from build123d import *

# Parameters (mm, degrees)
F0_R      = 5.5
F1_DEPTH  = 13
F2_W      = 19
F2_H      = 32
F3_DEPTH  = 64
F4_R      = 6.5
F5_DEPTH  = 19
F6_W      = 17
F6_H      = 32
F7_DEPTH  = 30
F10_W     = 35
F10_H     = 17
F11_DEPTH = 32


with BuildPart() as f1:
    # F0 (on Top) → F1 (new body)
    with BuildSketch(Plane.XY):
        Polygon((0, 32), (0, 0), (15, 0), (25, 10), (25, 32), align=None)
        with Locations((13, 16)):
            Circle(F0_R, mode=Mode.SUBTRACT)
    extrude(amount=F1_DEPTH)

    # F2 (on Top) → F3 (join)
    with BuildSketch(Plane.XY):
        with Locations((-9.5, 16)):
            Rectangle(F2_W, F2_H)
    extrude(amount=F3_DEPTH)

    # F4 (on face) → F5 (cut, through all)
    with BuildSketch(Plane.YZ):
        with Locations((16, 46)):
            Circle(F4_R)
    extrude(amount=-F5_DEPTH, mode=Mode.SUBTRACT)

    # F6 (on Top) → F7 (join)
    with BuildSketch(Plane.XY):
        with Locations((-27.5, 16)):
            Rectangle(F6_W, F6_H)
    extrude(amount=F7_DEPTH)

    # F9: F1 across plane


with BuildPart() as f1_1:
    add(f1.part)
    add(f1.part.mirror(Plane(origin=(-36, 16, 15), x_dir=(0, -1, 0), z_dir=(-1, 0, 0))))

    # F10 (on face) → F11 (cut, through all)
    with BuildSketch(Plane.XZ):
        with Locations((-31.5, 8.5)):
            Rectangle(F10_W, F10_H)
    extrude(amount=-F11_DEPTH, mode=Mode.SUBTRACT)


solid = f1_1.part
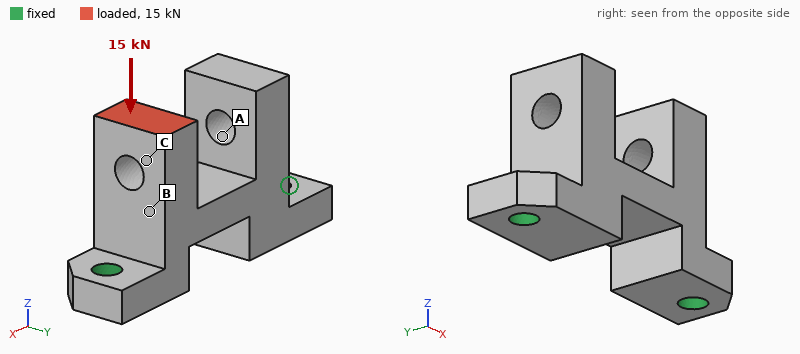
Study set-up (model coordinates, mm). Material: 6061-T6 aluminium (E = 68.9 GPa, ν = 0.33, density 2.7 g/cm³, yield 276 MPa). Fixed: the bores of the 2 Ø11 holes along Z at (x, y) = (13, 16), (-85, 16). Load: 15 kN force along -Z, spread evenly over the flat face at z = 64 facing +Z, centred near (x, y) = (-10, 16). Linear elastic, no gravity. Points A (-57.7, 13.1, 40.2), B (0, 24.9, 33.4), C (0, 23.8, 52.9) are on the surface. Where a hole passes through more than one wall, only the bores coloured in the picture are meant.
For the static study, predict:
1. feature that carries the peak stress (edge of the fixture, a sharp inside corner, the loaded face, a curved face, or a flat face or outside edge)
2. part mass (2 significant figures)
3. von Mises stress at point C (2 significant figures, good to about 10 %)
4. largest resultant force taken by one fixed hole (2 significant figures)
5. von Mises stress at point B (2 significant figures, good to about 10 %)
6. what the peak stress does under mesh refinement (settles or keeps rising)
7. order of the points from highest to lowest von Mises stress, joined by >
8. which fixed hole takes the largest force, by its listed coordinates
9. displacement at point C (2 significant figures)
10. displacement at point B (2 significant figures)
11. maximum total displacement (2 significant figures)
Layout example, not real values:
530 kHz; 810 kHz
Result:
edge of the fixture; 280 g; 49 MPa; 14 kN; 34 MPa; keeps rising; C > B > A; (13, 16); 61 µm; 50 µm; 69 µm
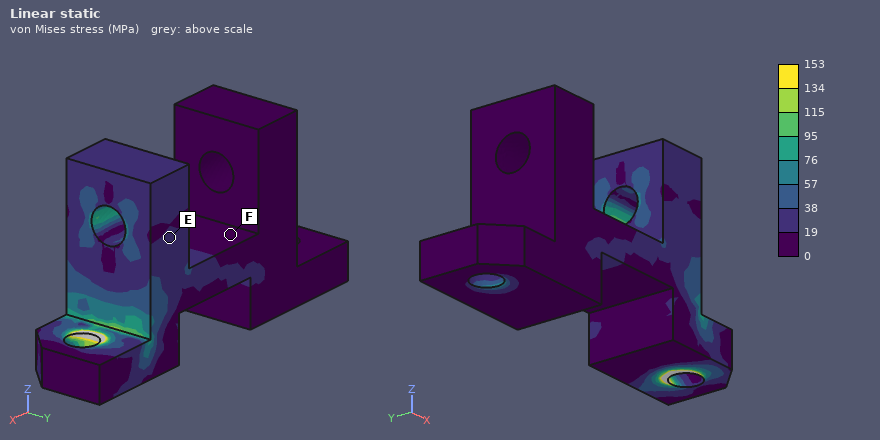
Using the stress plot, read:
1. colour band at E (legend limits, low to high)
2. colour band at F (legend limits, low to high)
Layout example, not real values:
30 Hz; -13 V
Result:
19 to 38 MPa; 0 to 19 MPa
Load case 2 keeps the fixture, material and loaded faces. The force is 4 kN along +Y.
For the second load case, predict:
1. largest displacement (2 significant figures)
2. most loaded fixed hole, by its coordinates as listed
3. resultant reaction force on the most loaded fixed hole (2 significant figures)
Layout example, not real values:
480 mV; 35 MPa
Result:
0.35 mm; (13, 16); 3.0 kN
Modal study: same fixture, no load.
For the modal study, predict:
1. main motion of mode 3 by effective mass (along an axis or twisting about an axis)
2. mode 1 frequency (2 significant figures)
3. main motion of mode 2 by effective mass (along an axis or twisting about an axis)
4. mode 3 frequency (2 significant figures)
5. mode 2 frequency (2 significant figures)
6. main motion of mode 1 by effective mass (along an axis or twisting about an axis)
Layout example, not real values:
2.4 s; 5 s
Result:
along X; 2600 Hz; twisting about Z; 5200 Hz; 4200 Hz; along Y
